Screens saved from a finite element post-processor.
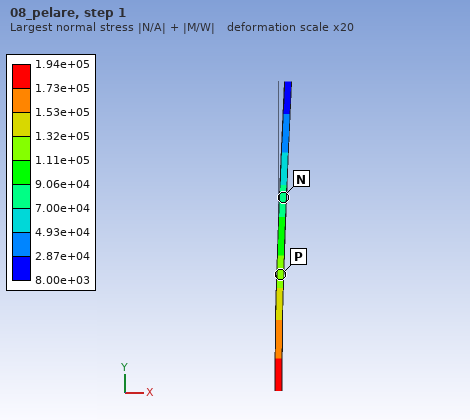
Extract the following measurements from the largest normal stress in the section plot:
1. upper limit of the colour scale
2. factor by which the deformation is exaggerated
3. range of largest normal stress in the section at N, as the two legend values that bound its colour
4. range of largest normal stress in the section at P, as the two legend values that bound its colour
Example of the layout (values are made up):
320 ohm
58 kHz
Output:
1.94e+05
20
7.00e+04 to 9.06e+04
1.11e+05 to 1.32e+05
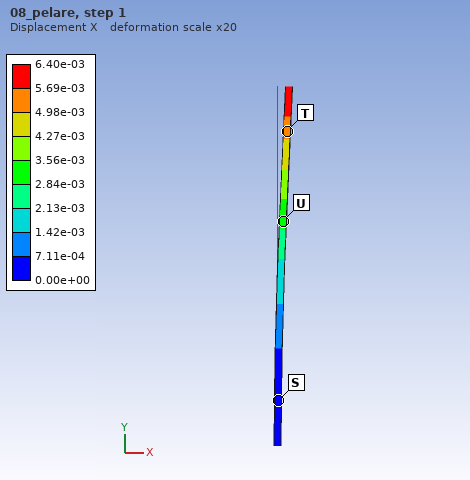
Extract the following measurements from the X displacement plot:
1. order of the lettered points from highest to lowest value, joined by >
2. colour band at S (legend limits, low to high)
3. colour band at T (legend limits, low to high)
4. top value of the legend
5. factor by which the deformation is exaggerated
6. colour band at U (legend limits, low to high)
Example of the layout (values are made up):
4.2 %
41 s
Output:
T > U > S
0.00e+00 to 7.11e-04
4.98e-03 to 5.69e-03
6.40e-03
20
2.84e-03 to 3.56e-03
